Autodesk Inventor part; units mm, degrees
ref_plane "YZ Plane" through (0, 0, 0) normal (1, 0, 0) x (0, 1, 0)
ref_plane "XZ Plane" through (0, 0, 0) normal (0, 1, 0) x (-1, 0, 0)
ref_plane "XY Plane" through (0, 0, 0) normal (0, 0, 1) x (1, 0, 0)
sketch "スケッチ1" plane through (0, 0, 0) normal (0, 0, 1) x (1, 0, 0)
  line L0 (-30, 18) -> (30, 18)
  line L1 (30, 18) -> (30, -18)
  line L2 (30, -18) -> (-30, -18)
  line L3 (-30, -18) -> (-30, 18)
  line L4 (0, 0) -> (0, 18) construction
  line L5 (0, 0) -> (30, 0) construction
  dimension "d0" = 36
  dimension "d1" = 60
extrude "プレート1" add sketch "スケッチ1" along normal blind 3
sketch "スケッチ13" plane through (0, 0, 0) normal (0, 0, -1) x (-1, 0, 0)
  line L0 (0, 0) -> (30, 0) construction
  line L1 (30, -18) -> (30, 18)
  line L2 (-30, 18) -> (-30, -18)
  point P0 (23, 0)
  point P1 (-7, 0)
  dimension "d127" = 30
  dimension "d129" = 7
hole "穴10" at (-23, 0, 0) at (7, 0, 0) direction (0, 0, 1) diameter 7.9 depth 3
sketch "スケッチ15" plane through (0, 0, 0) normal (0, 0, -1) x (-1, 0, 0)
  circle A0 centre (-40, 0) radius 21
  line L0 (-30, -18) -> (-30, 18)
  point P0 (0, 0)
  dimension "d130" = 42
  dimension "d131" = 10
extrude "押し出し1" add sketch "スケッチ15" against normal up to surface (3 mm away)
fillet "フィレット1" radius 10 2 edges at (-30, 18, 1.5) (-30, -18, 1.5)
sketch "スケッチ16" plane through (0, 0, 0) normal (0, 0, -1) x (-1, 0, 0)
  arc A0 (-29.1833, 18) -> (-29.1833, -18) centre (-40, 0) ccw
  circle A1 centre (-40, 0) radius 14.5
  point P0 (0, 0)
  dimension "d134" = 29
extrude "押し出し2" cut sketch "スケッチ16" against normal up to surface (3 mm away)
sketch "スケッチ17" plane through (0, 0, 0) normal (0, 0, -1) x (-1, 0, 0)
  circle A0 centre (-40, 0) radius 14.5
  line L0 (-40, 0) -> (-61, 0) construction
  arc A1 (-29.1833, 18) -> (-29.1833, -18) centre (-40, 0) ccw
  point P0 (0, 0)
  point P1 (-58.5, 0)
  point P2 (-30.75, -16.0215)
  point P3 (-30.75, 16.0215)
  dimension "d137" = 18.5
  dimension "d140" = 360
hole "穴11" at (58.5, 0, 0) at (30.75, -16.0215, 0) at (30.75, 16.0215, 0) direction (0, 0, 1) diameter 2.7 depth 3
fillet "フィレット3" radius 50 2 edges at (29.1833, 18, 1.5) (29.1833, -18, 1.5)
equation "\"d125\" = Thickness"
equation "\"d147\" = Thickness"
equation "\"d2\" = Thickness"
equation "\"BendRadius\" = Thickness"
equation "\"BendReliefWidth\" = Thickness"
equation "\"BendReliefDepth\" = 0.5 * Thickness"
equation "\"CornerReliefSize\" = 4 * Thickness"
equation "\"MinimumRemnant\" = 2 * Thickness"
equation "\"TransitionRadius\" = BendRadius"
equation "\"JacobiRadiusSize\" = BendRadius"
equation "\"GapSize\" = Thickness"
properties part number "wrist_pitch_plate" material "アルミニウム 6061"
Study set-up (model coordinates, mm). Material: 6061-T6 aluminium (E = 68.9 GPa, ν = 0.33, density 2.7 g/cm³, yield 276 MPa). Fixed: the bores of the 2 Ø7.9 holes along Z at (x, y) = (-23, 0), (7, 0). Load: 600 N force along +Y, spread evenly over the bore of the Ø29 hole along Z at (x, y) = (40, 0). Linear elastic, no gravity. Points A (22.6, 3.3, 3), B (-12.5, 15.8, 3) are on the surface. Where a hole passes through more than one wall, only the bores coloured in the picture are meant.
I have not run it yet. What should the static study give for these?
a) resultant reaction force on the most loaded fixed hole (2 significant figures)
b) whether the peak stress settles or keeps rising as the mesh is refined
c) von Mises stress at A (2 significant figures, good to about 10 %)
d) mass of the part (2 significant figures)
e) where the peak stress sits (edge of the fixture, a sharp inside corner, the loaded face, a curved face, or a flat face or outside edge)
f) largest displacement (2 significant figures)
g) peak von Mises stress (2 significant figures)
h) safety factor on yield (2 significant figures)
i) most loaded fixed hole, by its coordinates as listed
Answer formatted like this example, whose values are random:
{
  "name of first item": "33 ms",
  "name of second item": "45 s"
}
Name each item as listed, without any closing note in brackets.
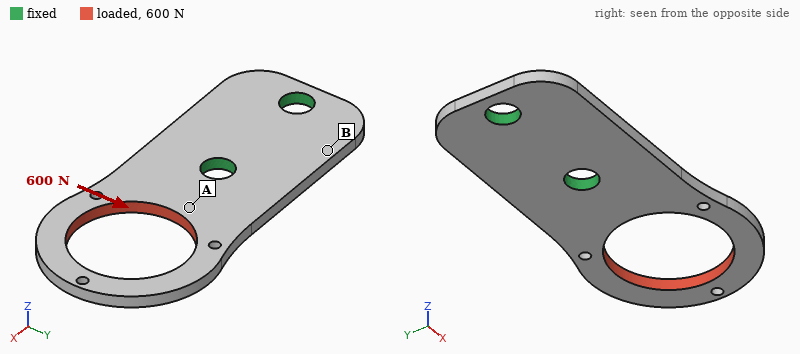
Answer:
{
  "resultant reaction force on the most loaded fixed hole": "1.0 kN",
  "whether the peak stress settles or keeps rising as the mesh is refined": "settles",
  "von Mises stress at A": "26 MPa",
  "mass of the part": "20 g",
  "where the peak stress sits": "a curved face",
  "largest displacement": "0.12 mm",
  "peak von Mises stress": "91 MPa",
  "safety factor on yield": "3.0",
  "most loaded fixed hole, by its coordinates as listed": "(7, 0)"
}
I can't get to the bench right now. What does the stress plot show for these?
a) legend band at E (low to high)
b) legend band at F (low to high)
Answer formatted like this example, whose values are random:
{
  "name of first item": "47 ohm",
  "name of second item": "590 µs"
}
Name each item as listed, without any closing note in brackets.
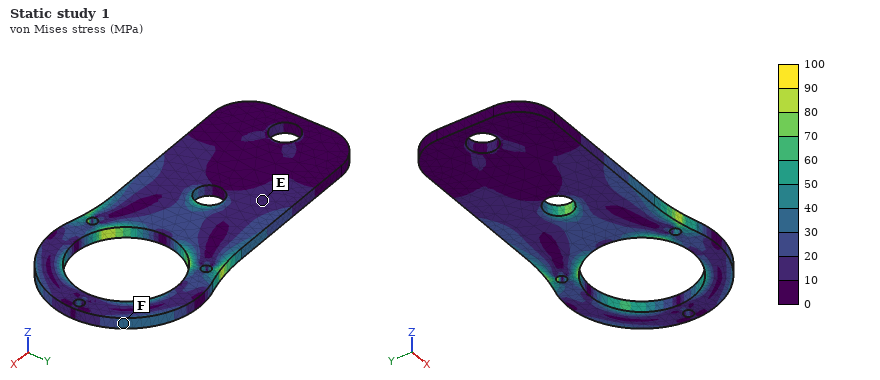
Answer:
{
  "legend band at E": "10 to 20 MPa",
  "legend band at F": "30 to 40 MPa"
}
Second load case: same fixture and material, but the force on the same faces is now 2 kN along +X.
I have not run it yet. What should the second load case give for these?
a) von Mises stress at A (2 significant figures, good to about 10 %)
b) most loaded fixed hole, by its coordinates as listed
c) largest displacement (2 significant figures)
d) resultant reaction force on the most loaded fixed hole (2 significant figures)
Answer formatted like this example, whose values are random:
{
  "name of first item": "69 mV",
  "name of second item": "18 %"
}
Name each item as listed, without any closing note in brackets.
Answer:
{
  "von Mises stress at A": "22 MPa",
  "most loaded fixed hole, by its coordinates as listed": "(7, 0)",
  "largest displacement": "63 µm",
  "resultant reaction force on the most loaded fixed hole": "1.6 kN"
}
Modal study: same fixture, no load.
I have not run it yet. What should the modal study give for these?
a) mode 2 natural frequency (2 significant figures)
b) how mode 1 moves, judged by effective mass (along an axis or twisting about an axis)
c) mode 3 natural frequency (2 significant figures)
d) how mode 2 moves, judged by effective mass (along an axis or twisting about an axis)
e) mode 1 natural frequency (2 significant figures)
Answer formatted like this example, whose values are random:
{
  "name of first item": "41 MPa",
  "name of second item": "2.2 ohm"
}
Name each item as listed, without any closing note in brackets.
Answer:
{
  "mode 2 natural frequency": "2300 Hz",
  "how mode 1 moves, judged by effective mass": "along Z",
  "mode 3 natural frequency": "4700 Hz",
  "how mode 2 moves, judged by effective mass": "twisting about X",
  "mode 1 natural frequency": "1000 Hz"
}
